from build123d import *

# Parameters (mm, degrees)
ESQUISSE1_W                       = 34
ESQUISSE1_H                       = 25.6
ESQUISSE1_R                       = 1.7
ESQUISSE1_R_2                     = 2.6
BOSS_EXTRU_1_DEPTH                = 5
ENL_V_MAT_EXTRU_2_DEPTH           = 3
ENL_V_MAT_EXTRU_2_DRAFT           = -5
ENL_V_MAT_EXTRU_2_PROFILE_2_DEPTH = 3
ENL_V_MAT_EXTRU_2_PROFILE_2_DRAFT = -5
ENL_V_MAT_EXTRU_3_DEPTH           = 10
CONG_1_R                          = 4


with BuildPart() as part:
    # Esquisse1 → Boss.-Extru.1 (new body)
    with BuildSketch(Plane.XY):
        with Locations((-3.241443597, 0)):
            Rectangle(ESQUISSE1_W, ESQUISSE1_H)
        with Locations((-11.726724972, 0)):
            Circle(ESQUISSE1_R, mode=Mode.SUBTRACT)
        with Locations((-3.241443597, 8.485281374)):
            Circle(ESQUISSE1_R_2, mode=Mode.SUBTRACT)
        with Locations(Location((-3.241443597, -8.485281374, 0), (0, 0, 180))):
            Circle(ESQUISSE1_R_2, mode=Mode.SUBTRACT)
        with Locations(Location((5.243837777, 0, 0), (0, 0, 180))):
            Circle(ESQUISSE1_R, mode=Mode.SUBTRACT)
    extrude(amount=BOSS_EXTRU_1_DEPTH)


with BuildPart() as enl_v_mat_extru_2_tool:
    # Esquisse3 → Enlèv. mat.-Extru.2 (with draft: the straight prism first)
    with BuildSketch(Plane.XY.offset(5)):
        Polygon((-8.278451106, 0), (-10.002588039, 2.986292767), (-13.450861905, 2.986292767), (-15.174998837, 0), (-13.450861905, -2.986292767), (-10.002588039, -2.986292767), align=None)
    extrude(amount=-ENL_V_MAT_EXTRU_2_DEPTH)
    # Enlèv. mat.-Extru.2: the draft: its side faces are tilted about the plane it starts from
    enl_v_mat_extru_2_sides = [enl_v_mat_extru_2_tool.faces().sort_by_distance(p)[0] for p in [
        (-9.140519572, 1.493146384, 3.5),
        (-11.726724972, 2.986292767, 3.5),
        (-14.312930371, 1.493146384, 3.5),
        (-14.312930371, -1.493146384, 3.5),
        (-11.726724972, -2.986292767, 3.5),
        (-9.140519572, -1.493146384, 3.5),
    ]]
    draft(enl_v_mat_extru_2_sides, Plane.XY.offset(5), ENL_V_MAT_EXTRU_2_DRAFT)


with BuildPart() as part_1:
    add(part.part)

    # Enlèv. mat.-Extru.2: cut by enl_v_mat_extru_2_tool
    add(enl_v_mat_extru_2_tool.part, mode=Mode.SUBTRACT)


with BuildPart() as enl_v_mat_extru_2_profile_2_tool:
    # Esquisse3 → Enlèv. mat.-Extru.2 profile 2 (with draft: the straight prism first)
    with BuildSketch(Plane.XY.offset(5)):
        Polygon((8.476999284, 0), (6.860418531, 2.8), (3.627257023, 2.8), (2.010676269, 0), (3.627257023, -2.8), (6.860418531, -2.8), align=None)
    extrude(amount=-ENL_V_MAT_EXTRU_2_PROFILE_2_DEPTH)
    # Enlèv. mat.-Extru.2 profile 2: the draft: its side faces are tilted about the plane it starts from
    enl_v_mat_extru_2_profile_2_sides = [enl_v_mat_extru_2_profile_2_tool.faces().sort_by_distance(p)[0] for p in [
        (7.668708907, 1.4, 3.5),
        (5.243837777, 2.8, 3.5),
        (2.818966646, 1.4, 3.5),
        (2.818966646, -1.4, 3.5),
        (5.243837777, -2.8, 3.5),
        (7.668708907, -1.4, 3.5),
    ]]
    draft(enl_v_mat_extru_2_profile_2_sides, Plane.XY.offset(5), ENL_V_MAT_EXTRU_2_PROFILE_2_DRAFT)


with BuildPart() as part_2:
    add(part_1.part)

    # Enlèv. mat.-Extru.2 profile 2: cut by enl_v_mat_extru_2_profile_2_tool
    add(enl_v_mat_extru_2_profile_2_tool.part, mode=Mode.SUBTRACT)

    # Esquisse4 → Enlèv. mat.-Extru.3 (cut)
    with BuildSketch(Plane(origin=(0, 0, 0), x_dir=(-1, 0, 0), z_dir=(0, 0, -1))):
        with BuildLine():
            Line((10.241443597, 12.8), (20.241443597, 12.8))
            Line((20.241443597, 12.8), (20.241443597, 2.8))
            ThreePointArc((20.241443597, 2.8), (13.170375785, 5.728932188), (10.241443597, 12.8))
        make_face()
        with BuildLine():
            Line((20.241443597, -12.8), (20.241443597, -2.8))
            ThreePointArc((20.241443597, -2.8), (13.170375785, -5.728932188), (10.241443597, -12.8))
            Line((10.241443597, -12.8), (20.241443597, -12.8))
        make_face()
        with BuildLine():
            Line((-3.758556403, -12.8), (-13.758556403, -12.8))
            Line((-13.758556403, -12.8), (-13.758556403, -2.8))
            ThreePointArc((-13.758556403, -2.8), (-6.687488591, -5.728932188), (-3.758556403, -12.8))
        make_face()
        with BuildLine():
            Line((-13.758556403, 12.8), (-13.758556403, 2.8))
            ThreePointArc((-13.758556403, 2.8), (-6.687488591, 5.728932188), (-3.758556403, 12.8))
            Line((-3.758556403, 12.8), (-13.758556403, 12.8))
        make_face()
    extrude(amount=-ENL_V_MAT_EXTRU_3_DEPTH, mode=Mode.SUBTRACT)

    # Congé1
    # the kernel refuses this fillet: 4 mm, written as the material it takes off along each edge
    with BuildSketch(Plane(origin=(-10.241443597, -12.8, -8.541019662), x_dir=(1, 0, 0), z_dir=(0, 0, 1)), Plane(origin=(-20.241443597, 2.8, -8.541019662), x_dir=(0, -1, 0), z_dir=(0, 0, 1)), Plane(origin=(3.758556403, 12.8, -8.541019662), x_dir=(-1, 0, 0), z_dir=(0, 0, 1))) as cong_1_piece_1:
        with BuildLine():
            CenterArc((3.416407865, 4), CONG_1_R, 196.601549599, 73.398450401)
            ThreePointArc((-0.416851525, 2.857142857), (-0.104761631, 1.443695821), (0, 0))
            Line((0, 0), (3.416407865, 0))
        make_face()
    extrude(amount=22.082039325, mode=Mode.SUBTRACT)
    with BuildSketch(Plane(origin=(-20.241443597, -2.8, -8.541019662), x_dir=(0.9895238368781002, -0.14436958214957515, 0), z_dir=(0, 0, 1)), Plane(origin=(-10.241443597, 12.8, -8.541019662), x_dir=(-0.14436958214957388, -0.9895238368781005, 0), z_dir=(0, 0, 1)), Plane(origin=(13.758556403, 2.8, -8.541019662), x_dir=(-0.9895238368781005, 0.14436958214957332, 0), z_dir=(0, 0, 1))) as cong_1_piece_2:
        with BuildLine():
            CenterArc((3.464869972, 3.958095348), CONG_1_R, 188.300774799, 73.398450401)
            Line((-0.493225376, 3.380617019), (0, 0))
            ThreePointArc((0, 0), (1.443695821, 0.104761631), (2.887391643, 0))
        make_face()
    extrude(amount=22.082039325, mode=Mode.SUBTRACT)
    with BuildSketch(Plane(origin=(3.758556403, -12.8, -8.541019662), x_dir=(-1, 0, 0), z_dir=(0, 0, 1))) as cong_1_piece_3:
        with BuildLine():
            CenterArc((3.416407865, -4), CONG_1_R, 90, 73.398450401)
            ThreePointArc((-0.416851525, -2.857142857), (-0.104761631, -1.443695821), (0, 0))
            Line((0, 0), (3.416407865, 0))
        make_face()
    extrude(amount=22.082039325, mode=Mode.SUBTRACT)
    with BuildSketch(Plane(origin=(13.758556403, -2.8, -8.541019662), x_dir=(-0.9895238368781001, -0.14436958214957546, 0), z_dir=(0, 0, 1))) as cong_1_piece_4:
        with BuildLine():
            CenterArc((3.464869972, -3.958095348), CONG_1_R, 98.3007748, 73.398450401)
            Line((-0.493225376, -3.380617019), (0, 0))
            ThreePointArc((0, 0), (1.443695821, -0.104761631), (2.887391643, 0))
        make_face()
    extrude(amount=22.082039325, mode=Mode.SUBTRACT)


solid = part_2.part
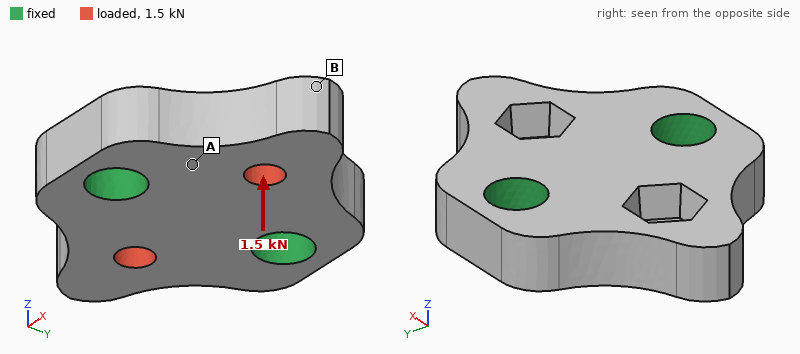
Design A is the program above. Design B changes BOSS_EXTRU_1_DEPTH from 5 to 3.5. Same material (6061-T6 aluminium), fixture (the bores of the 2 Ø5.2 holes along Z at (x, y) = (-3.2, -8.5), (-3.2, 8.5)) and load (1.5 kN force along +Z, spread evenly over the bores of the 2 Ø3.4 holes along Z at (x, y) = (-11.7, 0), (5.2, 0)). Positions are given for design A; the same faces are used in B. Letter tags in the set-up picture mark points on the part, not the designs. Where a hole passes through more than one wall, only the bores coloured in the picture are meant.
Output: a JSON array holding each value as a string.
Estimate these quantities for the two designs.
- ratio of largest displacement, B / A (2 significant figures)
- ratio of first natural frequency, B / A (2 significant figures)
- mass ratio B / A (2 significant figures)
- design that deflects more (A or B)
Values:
["2.5", "0.76", "0.71", "B"]
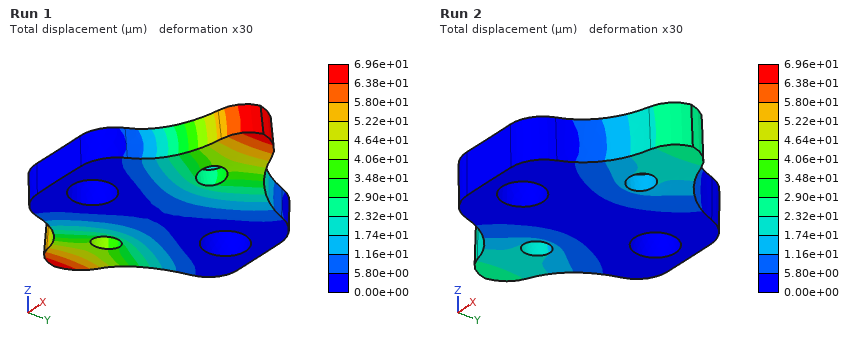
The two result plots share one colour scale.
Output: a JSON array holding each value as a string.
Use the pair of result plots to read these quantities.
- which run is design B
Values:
["Run 1"]
